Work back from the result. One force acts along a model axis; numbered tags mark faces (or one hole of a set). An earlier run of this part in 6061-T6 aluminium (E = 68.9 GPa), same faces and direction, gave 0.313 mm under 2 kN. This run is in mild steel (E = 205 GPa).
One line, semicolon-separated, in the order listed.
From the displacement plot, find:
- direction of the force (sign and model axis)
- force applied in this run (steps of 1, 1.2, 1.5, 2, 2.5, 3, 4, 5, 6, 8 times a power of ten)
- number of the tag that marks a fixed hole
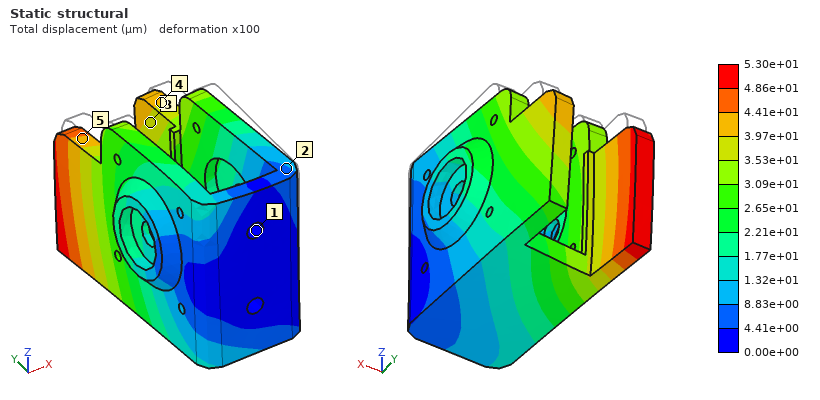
-Z; 1 kN; 1
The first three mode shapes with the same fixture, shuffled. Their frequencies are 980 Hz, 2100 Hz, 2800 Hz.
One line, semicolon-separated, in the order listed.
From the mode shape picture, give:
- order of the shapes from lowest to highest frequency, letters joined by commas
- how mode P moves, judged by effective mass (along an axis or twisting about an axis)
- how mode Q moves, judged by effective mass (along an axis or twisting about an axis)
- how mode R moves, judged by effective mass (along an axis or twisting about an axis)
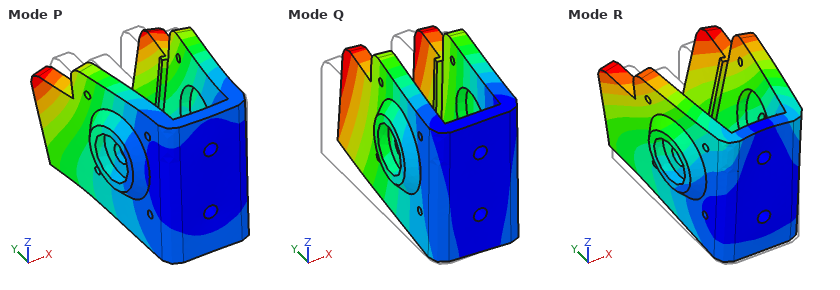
Q, R, P; along Z; along X; along Z
